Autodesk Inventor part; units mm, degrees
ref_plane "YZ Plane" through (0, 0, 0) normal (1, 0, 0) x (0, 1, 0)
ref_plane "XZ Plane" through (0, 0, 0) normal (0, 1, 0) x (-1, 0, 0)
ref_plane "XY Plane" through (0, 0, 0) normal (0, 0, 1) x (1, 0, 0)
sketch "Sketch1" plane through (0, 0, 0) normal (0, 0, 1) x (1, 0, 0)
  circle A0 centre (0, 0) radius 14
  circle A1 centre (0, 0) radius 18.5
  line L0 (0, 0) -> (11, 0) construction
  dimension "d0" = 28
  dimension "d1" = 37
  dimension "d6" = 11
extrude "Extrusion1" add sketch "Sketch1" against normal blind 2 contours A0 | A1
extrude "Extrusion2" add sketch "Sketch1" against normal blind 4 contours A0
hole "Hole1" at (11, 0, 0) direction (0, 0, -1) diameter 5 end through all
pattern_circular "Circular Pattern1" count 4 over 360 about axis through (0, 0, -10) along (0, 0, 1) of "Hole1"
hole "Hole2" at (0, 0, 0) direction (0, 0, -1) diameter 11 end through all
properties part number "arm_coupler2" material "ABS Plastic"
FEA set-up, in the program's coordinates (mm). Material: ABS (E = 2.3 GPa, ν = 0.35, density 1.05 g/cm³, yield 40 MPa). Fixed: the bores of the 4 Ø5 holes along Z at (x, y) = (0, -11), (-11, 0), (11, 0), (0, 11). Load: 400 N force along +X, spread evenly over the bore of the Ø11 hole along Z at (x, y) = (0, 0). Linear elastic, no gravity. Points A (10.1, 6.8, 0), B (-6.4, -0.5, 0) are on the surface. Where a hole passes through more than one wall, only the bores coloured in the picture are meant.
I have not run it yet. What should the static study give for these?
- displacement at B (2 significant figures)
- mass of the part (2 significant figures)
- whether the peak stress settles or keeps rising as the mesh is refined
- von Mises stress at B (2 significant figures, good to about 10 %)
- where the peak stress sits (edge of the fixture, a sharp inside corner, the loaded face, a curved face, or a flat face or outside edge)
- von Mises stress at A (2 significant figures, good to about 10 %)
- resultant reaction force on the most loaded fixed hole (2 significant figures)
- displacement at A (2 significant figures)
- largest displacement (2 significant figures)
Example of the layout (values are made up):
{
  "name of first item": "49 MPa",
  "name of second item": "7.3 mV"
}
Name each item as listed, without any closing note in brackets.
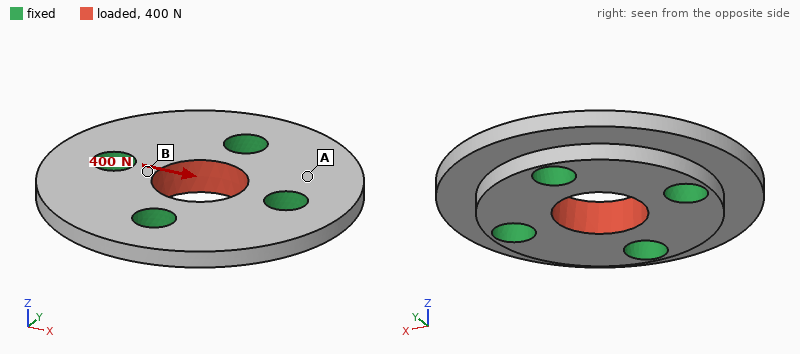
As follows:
{
  "displacement at B": "3.4 µm",
  "mass of the part": "2.8 g",
  "whether the peak stress settles or keeps rising as the mesh is refined": "keeps rising",
  "von Mises stress at B": "3.6 MPa",
  "where the peak stress sits": "edge of the fixture",
  "von Mises stress at A": "1.1 MPa",
  "resultant reaction force on the most loaded fixed hole": "120 N",
  "displacement at A": "3.9 µm",
  "largest displacement": "10 µm"
}
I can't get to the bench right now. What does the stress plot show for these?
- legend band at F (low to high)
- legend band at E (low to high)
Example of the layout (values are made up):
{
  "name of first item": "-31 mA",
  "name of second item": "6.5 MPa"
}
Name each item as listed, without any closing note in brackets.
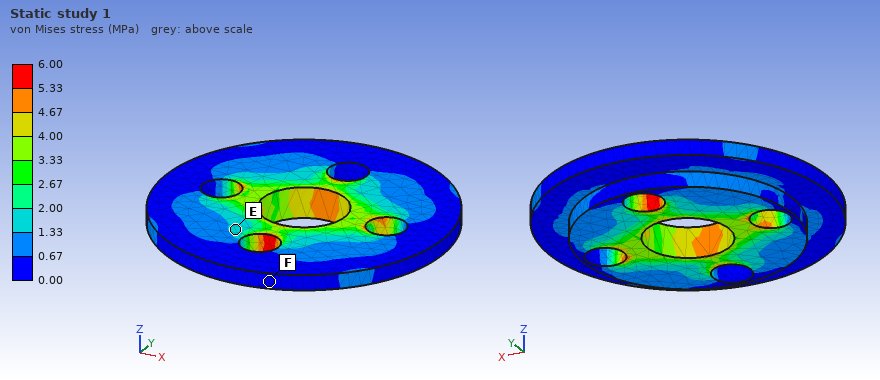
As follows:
{
  "legend band at F": "0.00 to 0.67 MPa",
  "legend band at E": "1.33 to 2.00 MPa"
}
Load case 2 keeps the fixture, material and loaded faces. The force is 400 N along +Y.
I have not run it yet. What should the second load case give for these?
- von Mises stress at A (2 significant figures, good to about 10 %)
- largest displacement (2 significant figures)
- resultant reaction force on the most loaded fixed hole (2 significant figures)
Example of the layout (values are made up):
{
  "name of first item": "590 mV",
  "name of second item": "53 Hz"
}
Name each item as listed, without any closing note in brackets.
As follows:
{
  "von Mises stress at A": "1.0 MPa",
  "largest displacement": "10 µm",
  "resultant reaction force on the most loaded fixed hole": "120 N"
}
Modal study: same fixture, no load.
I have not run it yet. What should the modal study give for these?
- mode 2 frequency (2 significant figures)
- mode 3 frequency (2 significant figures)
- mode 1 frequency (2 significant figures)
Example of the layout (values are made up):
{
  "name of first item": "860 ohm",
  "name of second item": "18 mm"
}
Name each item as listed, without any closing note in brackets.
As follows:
{
  "mode 2 frequency": "11 kHz",
  "mode 3 frequency": "11 kHz",
  "mode 1 frequency": "11 kHz"
}
